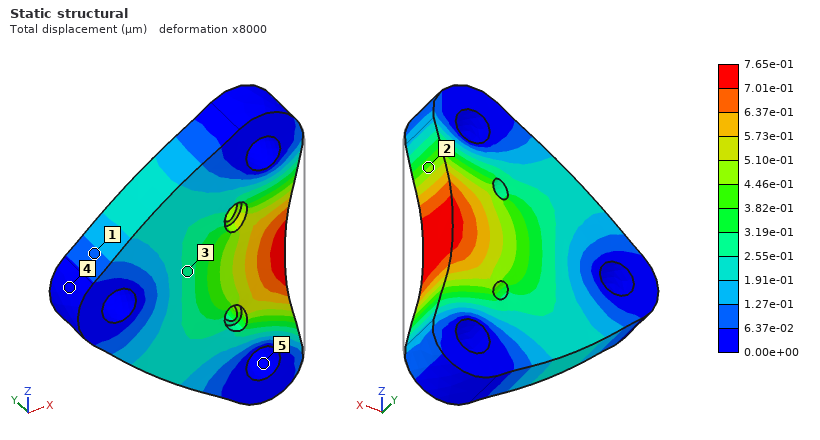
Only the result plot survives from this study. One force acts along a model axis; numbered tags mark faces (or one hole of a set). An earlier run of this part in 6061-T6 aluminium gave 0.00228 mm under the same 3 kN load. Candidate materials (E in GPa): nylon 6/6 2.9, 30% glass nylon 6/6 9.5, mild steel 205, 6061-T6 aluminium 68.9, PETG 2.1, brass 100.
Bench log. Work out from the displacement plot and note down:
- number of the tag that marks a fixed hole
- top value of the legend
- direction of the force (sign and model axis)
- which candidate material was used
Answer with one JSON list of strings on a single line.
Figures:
["5", "7.65e-01 µm", "-X", "mild steel"]
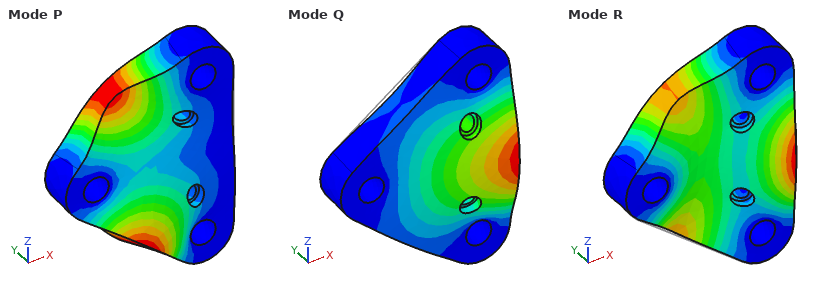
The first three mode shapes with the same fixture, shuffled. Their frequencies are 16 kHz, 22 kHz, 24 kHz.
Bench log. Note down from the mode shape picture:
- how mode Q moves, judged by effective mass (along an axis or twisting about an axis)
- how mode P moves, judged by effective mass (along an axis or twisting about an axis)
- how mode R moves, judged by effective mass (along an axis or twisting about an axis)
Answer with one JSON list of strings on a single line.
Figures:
["along Y", "twisting about X", "along Y"]
